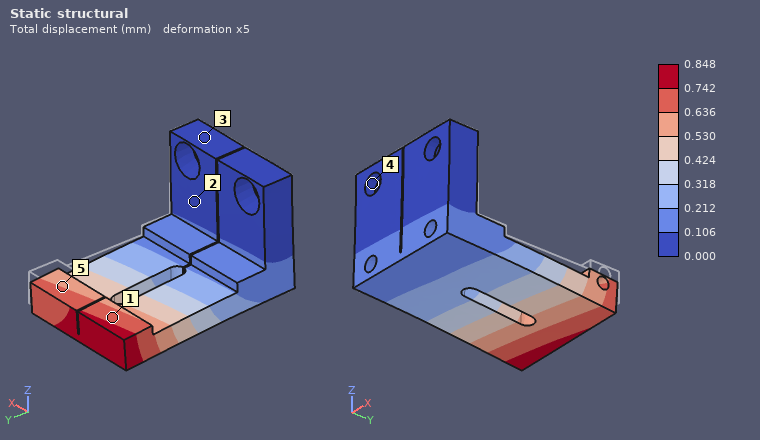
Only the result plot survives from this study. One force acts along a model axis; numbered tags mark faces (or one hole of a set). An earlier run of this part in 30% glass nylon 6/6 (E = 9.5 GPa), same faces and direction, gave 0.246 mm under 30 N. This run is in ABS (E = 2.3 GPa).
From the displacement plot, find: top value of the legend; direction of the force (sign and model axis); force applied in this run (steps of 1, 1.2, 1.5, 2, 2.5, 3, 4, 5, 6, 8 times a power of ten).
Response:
0.848 mm
-Z
25 N
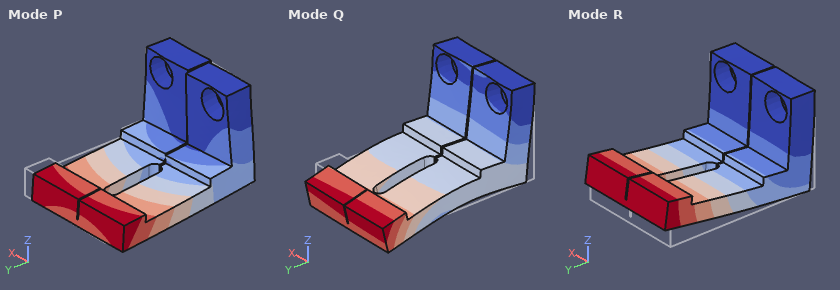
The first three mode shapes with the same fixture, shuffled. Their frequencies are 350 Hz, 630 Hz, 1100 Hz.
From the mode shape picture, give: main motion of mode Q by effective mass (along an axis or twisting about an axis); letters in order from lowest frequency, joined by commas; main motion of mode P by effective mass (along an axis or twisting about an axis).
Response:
along Y
R, P, Q
along X
